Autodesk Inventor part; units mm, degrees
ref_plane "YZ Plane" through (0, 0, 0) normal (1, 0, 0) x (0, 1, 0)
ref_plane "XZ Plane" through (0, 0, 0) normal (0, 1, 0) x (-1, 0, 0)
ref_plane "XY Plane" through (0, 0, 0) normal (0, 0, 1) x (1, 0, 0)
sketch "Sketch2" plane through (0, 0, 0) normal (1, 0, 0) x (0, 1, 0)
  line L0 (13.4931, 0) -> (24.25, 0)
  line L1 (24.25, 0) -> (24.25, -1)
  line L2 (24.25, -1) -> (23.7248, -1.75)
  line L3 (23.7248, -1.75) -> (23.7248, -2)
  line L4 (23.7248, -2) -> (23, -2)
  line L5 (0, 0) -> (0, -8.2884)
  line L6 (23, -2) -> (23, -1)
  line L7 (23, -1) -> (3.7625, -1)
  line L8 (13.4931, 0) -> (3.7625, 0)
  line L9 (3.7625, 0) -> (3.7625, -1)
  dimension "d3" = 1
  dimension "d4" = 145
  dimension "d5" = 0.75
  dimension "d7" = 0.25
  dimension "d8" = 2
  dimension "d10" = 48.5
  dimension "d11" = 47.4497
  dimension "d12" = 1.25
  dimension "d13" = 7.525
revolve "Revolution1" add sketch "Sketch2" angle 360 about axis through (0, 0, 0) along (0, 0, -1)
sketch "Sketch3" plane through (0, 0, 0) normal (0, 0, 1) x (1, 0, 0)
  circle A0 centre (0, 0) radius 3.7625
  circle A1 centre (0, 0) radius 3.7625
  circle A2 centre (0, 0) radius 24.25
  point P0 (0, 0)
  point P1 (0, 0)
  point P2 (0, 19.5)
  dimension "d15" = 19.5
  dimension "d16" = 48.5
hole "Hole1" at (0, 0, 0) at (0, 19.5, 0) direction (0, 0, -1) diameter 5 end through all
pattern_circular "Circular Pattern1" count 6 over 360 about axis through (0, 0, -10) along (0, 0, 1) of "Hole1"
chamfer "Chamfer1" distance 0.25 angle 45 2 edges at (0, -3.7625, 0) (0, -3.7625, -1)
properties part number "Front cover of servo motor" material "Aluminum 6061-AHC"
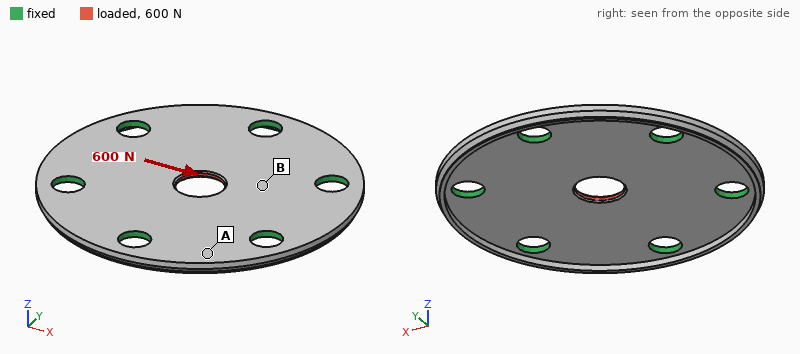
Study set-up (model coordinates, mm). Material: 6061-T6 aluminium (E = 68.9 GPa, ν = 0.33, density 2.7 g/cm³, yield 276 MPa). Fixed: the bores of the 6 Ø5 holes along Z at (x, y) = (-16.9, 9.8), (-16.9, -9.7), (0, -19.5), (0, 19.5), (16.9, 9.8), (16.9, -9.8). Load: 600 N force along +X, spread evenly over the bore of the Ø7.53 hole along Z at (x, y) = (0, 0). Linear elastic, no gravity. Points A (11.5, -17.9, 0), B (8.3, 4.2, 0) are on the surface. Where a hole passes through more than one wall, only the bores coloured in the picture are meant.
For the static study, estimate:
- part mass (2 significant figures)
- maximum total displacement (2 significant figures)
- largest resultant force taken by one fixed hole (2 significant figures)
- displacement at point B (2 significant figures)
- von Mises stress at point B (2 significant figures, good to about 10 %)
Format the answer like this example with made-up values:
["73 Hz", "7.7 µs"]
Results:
["4.9 g", "4.1 µm", "140 N", "2.0 µm", "17 MPa"]
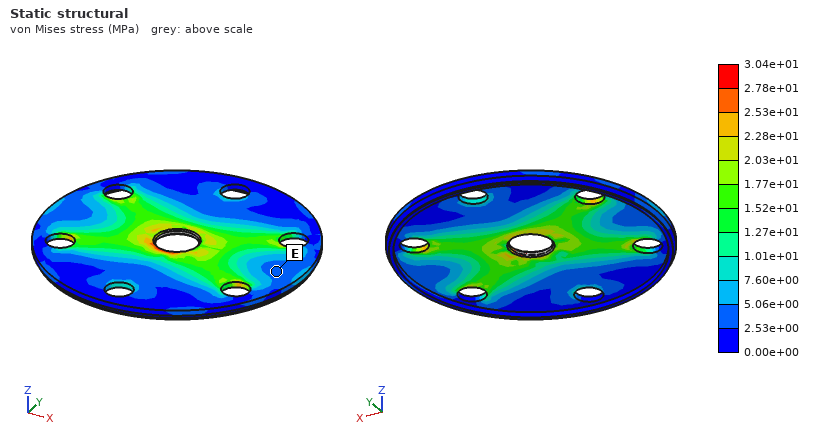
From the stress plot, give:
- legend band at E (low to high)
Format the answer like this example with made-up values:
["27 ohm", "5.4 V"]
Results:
["2.53e+00 to 5.06e+00 MPa"]
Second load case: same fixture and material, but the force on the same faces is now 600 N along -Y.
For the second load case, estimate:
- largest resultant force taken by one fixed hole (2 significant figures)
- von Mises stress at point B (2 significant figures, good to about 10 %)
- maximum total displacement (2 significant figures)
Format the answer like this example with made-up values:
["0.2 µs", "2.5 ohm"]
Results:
["160 N", "11 MPa", "4.1 µm"]
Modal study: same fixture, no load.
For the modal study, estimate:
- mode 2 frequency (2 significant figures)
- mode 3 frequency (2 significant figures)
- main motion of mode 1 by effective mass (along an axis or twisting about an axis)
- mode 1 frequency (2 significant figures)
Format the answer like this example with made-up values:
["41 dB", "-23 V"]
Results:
["14 kHz", "14 kHz", "along Z", "7400 Hz"]
